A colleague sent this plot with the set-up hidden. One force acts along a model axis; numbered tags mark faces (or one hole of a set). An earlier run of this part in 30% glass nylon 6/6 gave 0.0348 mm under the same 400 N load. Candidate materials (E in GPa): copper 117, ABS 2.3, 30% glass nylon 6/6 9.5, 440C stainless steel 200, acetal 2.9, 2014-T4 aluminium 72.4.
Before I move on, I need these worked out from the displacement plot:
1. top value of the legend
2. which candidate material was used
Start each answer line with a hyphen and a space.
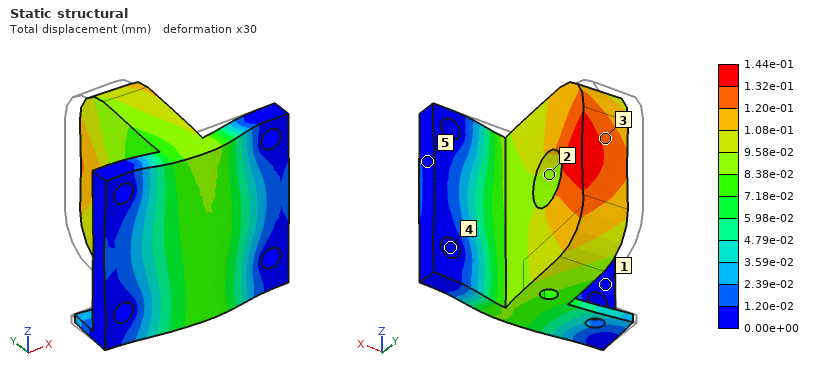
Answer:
- 1.44e-01 mm
- ABS
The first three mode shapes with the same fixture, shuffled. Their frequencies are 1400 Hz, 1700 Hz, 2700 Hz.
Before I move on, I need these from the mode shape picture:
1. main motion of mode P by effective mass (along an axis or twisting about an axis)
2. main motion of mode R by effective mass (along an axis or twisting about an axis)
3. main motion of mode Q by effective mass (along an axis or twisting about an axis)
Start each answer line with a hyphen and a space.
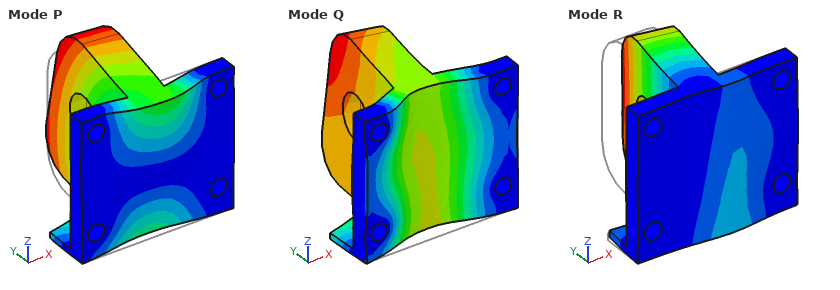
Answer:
- along Z
- along X
- along Y
